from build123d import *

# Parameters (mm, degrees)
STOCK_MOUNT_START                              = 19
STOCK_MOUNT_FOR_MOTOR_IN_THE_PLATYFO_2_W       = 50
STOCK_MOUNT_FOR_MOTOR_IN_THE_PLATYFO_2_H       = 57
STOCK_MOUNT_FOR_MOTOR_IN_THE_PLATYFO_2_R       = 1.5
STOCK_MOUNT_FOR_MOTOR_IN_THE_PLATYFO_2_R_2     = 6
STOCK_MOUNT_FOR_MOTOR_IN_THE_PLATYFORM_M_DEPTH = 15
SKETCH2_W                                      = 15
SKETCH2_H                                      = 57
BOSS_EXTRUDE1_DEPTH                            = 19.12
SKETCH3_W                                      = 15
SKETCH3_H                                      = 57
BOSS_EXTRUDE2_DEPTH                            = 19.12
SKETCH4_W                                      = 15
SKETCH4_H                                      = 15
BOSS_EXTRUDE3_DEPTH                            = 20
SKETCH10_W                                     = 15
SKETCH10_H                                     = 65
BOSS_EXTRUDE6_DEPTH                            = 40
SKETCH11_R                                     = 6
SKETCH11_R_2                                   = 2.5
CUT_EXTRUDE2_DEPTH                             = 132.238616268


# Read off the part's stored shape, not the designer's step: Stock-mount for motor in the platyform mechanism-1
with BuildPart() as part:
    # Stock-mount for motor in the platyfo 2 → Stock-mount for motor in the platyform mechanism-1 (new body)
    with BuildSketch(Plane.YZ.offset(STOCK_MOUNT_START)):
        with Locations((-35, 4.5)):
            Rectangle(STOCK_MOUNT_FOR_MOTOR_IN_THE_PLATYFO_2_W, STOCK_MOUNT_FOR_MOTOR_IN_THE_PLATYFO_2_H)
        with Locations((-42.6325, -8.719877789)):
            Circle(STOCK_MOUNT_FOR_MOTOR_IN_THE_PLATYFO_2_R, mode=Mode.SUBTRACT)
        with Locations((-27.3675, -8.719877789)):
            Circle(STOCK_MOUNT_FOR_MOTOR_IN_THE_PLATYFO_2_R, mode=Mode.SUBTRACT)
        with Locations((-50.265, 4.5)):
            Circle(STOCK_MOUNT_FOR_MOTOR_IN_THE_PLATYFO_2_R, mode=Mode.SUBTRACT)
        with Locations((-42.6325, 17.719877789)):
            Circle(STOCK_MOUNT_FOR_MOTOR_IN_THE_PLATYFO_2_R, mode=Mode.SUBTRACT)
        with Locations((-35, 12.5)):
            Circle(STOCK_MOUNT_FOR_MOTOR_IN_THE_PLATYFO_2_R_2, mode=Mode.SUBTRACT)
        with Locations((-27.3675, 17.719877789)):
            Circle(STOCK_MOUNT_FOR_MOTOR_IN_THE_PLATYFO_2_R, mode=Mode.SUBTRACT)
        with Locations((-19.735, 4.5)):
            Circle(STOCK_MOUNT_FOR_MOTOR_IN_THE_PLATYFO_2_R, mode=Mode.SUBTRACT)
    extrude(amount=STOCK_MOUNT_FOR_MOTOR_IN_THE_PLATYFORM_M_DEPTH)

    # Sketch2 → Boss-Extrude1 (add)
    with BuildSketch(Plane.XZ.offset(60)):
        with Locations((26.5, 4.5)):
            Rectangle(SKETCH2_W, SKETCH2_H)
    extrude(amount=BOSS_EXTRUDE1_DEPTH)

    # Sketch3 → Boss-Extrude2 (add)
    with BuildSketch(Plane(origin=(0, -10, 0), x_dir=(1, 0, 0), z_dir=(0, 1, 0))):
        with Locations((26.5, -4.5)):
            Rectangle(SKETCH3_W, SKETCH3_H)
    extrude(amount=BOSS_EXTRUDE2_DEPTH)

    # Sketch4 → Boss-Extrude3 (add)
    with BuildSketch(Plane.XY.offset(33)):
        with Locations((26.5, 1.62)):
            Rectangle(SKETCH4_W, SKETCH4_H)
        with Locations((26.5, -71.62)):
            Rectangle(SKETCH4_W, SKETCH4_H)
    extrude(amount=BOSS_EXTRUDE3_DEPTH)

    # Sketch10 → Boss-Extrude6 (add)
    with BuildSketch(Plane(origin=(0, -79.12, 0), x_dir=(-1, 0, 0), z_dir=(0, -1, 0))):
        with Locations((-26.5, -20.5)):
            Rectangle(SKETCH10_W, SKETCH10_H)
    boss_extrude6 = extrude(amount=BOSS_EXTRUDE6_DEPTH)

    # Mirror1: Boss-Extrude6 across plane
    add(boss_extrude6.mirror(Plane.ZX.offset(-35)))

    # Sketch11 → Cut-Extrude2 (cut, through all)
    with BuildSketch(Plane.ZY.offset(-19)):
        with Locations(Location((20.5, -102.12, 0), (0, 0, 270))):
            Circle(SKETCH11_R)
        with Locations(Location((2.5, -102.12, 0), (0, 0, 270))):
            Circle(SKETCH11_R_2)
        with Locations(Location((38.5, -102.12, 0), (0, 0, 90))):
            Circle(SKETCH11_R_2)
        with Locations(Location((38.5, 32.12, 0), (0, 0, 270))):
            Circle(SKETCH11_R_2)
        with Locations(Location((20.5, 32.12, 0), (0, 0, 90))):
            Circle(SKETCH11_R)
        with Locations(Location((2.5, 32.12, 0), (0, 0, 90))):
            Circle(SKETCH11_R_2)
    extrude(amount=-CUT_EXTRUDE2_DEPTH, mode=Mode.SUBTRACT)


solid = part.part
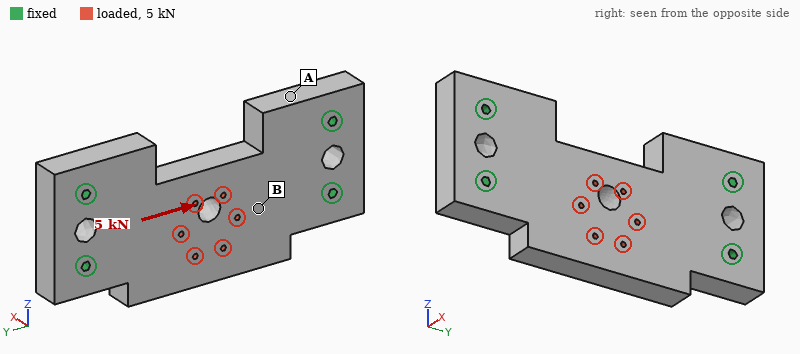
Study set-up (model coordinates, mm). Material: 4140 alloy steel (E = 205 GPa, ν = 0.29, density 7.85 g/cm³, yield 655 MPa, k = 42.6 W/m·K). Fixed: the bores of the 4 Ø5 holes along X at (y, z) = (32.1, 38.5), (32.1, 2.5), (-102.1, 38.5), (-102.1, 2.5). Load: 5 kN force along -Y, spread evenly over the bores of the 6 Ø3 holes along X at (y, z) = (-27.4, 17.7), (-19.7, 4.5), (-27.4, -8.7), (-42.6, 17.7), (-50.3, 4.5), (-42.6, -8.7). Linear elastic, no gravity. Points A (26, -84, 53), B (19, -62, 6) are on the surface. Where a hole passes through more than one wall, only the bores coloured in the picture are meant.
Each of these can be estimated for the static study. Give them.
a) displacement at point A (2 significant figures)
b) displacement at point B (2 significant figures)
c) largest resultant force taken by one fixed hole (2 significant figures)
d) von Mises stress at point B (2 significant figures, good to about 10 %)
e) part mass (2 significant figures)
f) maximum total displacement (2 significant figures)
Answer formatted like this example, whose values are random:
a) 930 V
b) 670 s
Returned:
a) 0.19 µm
b) 0.83 µm
c) 1.6 kN
d) 4.2 MPa
e) 1.2 kg
f) 1.3 µm
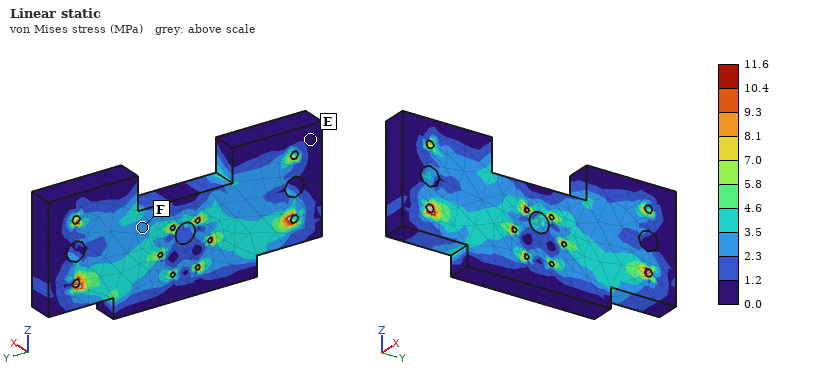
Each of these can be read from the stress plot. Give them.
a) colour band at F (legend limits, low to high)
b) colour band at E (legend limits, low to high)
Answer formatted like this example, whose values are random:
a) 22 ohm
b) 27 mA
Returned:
a) 2.3 to 3.5 MPa
b) 0.0 to 1.2 MPa
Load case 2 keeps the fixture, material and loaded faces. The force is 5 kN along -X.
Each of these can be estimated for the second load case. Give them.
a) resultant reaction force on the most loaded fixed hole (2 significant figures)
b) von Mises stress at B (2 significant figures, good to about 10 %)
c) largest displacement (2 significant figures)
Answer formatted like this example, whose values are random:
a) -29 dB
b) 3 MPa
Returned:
a) 2.1 kN
b) 9.3 MPa
c) 32 µm
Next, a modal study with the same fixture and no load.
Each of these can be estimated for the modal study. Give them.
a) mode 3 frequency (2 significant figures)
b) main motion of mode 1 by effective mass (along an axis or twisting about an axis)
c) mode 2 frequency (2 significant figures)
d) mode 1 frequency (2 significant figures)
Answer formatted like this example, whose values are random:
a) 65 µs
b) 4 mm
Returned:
a) 8600 Hz
b) along X
c) 6100 Hz
d) 3400 Hz
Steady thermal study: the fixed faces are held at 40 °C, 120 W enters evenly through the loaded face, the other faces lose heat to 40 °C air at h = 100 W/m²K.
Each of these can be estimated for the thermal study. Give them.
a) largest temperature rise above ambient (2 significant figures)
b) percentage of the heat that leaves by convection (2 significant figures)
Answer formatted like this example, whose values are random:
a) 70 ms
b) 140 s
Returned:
a) 68 K
b) 57 %
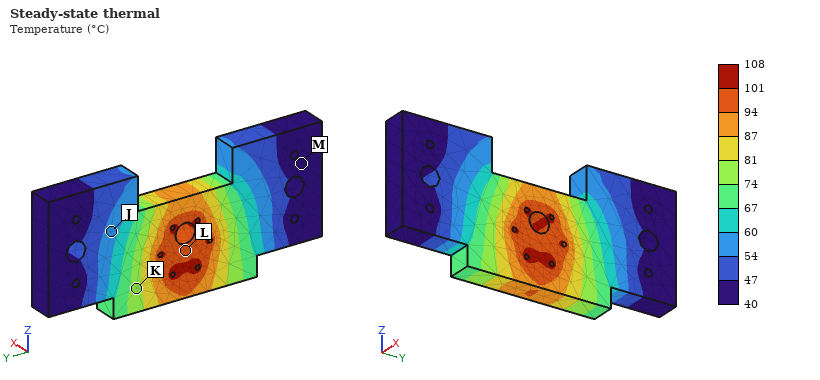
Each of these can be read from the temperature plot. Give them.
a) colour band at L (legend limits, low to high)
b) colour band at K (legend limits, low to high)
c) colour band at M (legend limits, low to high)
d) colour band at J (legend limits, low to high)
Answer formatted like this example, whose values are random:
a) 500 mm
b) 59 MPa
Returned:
a) 94 to 101 °C
b) 74 to 81 °C
c) 40 to 47 °C
d) 54 to 60 °C
